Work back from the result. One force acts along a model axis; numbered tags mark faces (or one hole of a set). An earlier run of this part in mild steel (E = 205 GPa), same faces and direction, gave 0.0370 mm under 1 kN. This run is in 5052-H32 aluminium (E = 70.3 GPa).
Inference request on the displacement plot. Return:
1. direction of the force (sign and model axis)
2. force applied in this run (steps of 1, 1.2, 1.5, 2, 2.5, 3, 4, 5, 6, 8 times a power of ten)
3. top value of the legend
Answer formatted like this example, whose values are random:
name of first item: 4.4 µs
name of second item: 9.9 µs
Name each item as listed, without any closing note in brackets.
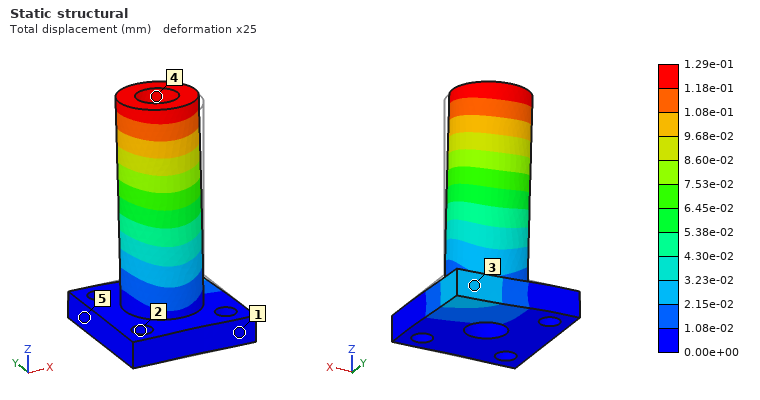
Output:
direction of the force: +Y
force applied in this run: 1.2 kN
top value of the legend: 1.29e-01 mm
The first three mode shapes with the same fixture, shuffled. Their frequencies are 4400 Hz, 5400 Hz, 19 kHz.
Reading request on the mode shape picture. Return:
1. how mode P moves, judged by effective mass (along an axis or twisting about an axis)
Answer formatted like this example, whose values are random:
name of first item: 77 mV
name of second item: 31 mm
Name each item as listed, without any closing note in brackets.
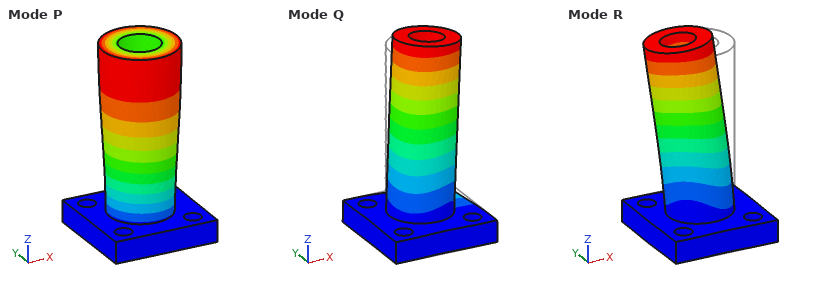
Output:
how mode P moves, judged by effective mass: twisting about Z
